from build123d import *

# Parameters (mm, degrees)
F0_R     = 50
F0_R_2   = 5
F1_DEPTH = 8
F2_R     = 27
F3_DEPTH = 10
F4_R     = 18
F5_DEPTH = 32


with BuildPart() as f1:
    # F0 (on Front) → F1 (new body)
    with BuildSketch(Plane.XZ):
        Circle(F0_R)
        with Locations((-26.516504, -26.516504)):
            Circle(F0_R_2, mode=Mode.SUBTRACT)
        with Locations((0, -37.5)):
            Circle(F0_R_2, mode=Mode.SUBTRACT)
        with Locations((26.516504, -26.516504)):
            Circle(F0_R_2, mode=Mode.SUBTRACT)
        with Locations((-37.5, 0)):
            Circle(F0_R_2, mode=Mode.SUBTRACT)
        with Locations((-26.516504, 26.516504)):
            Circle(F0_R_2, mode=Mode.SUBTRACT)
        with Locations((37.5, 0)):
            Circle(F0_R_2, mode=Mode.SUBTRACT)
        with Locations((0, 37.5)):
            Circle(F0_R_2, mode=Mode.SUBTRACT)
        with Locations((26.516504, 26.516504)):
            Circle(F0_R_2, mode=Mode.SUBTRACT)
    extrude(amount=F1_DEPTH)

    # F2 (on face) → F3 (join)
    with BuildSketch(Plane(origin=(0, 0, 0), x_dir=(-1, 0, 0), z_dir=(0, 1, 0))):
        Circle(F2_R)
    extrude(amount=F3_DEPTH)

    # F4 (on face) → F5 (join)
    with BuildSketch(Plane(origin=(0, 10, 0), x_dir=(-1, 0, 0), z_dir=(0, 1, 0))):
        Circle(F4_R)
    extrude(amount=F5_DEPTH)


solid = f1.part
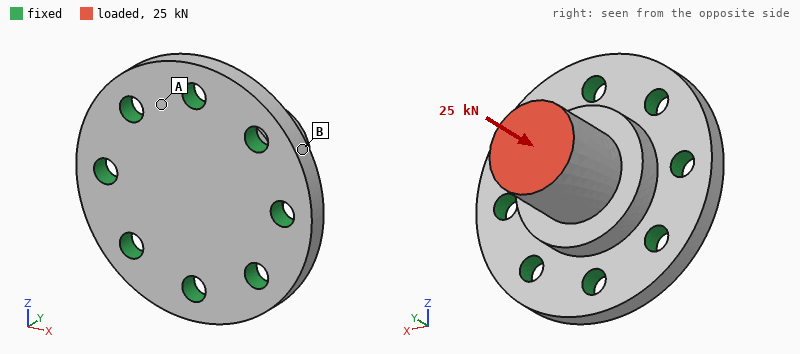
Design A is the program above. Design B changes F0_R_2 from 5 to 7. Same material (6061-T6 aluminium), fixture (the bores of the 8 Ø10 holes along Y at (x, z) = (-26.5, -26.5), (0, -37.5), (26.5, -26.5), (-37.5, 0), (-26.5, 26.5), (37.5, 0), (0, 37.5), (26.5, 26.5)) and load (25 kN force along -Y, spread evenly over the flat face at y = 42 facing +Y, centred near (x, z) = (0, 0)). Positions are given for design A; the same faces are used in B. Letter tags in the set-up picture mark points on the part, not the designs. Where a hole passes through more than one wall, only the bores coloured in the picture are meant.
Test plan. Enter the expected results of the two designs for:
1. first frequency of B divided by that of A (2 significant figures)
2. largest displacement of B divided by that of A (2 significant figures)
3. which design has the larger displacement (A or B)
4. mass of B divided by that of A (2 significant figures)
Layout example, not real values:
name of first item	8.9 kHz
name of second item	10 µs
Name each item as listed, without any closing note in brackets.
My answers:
first frequency of B divided by that of A	1.1
largest displacement of B divided by that of A	0.84
which design has the larger displacement	A
mass of B divided by that of A	0.96
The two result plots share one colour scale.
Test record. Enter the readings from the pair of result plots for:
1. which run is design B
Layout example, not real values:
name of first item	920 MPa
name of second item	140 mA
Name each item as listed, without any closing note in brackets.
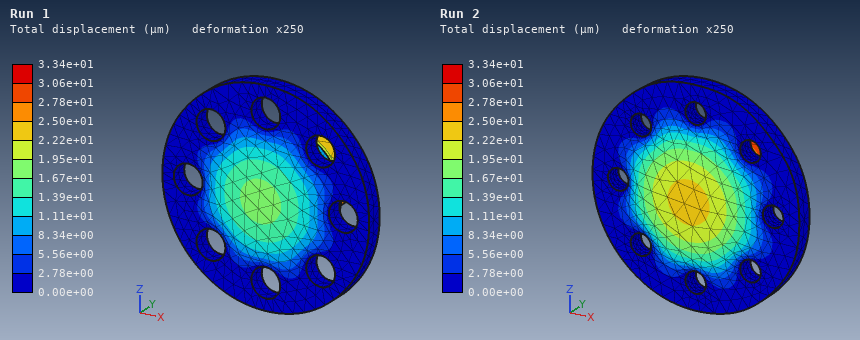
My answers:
which run is design B	Run 1
